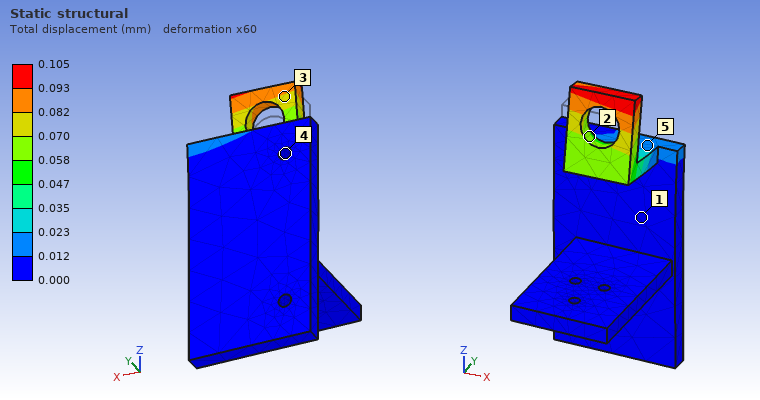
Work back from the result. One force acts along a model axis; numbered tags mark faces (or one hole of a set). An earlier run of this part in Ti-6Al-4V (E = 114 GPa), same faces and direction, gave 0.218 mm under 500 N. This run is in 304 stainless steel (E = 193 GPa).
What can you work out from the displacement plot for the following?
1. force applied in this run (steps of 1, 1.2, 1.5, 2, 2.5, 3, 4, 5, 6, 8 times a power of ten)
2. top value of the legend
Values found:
400 N
0.105 mm
